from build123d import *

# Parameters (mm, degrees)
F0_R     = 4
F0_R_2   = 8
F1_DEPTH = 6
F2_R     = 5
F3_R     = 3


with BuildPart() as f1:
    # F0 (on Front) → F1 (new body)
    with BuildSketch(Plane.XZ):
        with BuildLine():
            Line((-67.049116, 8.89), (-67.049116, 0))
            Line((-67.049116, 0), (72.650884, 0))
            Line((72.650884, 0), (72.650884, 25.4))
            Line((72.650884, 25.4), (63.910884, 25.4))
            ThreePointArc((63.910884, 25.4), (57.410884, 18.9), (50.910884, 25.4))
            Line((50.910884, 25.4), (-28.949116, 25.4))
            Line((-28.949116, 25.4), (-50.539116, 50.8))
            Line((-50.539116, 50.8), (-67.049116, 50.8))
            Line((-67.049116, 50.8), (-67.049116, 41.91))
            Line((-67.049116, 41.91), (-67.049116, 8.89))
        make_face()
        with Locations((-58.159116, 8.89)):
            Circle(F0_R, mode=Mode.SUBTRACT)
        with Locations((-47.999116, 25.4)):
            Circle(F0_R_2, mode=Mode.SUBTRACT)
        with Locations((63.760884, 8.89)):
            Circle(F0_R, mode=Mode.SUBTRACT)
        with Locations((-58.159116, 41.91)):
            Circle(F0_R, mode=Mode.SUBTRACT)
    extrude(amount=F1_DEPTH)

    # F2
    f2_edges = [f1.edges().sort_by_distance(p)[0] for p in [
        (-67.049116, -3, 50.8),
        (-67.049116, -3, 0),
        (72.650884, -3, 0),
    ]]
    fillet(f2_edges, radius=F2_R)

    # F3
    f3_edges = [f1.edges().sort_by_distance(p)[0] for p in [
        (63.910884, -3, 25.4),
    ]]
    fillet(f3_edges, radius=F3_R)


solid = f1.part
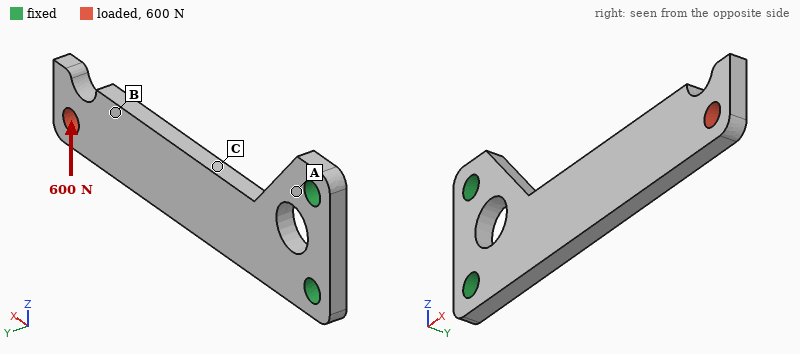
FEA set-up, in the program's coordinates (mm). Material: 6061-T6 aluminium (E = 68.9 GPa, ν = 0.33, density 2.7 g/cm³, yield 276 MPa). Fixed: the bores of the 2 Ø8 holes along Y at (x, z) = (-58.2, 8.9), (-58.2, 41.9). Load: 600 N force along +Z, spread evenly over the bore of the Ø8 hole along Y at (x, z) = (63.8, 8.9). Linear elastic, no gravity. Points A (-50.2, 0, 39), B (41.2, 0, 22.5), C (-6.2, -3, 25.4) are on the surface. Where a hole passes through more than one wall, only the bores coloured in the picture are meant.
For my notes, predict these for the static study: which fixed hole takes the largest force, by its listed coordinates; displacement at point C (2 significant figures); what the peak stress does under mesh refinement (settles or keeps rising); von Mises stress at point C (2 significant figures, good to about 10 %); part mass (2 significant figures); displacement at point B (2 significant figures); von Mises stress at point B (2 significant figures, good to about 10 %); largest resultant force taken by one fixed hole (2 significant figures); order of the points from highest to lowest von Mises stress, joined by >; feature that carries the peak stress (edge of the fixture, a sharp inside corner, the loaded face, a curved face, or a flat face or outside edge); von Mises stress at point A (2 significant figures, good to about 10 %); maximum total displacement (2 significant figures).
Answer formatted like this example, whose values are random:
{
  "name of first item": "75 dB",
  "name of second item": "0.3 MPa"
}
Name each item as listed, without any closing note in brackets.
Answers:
{
  "which fixed hole takes the largest force, by its listed coordinates": "(-58.2, 41.9)",
  "displacement at point C": "0.11 mm",
  "what the peak stress does under mesh refinement": "keeps rising",
  "von Mises stress at point C": "65 MPa",
  "part mass": "62 g",
  "displacement at point B": "0.36 mm",
  "von Mises stress at point B": "16 MPa",
  "largest resultant force taken by one fixed hole": "2.3 kN",
  "order of the points from highest to lowest von Mises stress, joined by >": "C > A > B",
  "feature that carries the peak stress": "a sharp inside corner",
  "von Mises stress at point A": "44 MPa",
  "maximum total displacement": "0.57 mm"
}
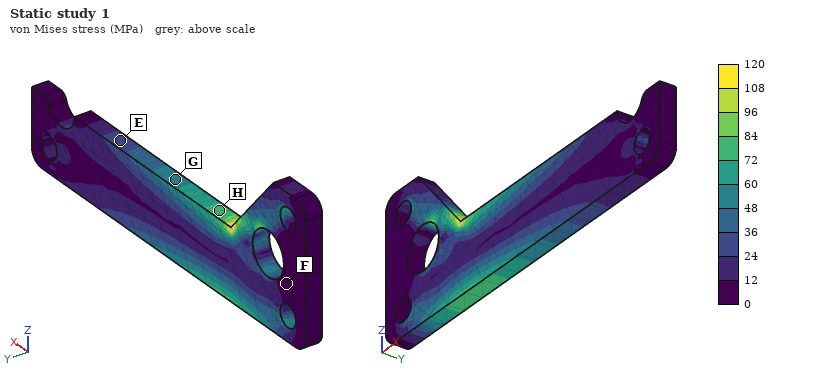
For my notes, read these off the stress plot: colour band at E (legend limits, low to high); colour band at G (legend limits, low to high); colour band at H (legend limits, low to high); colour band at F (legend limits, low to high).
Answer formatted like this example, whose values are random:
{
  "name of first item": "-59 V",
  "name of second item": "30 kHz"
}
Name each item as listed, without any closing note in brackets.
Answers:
{
  "colour band at E": "24 to 36 MPa",
  "colour band at G": "48 to 60 MPa",
  "colour band at H": "72 to 84 MPa",
  "colour band at F": "0 to 12 MPa"
}
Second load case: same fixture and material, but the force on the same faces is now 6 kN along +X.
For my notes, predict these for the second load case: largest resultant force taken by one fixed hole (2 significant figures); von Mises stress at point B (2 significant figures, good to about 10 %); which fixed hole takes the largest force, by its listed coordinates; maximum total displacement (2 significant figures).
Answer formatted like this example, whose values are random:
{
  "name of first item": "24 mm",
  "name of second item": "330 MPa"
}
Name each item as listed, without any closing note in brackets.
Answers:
{
  "largest resultant force taken by one fixed hole": "5.8 kN",
  "von Mises stress at point B": "11 MPa",
  "which fixed hole takes the largest force, by its listed coordinates": "(-58.2, 8.9)",
  "maximum total displacement": "0.32 mm"
}
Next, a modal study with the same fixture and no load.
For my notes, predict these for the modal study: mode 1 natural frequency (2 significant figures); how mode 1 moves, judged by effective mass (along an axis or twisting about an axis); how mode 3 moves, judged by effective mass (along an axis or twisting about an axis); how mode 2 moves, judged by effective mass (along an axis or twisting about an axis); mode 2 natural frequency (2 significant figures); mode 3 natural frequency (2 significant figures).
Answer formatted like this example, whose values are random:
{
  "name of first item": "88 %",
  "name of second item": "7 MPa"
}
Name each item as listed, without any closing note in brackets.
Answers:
{
  "mode 1 natural frequency": "320 Hz",
  "how mode 1 moves, judged by effective mass": "along Y",
  "how mode 3 moves, judged by effective mass": "along Y",
  "how mode 2 moves, judged by effective mass": "along Z",
  "mode 2 natural frequency": "1500 Hz",
  "mode 3 natural frequency": "1900 Hz"
}
